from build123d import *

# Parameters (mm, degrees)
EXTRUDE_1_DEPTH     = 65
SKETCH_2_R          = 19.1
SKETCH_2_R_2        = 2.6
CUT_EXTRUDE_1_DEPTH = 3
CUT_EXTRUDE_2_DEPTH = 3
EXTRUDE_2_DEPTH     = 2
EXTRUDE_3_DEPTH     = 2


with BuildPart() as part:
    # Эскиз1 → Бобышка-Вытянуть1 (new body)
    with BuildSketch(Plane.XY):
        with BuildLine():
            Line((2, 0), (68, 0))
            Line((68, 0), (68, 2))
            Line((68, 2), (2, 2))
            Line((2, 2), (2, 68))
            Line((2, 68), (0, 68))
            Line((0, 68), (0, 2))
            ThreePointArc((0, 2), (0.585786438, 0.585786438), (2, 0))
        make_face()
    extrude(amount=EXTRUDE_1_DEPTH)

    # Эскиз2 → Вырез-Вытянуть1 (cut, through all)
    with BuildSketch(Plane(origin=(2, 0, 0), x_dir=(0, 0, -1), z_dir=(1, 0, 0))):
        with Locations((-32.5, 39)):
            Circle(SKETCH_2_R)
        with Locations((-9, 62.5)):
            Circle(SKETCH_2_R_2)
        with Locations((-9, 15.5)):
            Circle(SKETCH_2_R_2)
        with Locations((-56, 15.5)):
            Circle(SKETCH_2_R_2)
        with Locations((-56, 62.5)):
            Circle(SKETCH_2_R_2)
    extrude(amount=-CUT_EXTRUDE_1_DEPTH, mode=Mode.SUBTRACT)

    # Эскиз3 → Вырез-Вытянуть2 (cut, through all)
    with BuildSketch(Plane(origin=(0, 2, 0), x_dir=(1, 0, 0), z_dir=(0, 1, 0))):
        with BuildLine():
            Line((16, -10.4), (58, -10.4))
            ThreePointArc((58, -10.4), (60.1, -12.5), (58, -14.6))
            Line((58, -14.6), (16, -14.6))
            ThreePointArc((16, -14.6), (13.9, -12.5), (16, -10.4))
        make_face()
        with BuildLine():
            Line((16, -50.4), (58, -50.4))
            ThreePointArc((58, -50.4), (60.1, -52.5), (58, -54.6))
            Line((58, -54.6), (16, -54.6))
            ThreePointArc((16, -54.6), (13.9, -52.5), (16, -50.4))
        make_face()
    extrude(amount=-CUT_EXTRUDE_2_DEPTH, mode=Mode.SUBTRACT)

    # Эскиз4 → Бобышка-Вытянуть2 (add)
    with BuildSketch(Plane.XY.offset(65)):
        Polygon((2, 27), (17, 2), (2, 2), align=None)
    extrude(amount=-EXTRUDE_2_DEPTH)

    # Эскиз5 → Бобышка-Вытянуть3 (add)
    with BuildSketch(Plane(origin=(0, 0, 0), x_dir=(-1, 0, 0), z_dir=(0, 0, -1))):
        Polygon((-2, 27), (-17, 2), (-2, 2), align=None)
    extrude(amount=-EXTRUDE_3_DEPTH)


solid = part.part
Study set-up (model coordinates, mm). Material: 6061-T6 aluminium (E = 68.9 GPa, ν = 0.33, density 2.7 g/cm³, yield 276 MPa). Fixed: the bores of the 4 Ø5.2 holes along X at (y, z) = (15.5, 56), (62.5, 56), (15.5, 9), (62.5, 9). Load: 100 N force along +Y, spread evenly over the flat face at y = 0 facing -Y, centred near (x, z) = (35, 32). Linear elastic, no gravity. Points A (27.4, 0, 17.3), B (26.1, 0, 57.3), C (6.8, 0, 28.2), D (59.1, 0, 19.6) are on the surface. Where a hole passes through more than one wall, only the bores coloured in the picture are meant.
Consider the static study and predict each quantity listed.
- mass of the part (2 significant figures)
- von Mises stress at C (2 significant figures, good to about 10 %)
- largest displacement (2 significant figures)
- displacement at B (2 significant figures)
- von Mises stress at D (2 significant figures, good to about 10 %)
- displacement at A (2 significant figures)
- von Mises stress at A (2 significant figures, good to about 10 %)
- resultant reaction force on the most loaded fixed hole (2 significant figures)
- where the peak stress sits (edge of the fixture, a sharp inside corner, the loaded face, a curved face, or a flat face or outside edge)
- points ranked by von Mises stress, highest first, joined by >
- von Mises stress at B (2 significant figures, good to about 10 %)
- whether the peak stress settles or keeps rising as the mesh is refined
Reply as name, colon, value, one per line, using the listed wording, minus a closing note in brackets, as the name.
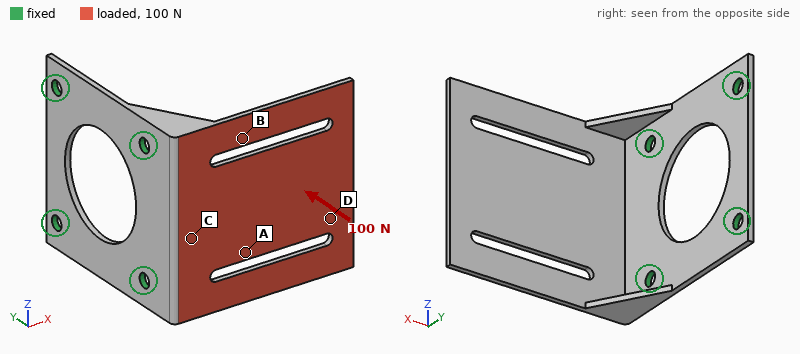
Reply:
mass of the part: 40 g
von Mises stress at C: 33 MPa
largest displacement: 1.3 mm
displacement at B: 0.22 mm
von Mises stress at D: 13 MPa
displacement at A: 0.33 mm
von Mises stress at A: 25 MPa
resultant reaction force on the most loaded fixed hole: 60 N
where the peak stress sits: a sharp inside corner
points ranked by von Mises stress, highest first, joined by >: B > C > A > D
von Mises stress at B: 53 MPa
whether the peak stress settles or keeps rising as the mesh is refined: keeps rising
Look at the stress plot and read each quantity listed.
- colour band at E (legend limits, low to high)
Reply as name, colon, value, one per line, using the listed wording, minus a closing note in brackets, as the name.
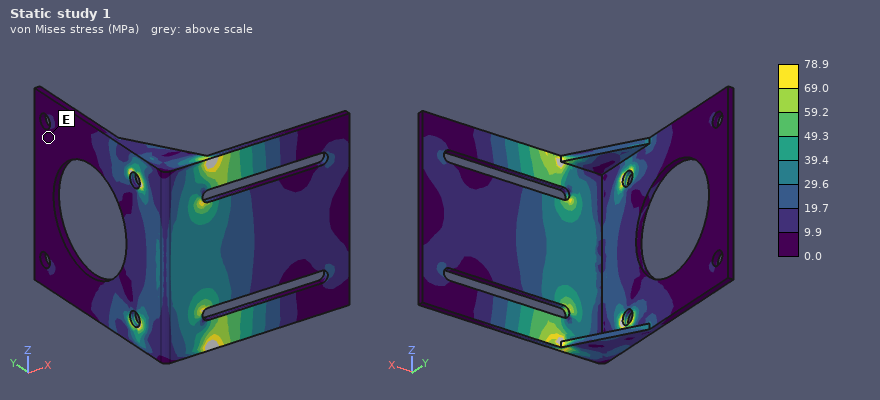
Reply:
colour band at E: 0.0 to 9.9 MPa
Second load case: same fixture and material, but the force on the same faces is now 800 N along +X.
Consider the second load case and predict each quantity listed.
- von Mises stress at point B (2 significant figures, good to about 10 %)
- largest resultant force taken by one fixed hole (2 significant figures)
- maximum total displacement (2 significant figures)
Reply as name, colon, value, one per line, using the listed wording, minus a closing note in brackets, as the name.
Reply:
von Mises stress at point B: 24 MPa
largest resultant force taken by one fixed hole: 440 N
maximum total displacement: 1.1 mm
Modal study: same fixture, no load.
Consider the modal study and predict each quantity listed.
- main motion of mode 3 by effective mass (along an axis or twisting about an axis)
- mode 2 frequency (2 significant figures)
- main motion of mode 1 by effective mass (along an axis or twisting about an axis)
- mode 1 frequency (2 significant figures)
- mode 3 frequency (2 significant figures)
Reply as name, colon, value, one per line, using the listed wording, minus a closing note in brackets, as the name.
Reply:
main motion of mode 3 by effective mass: along Z
mode 2 frequency: 990 Hz
main motion of mode 1 by effective mass: along Y
mode 1 frequency: 380 Hz
mode 3 frequency: 1600 Hz
